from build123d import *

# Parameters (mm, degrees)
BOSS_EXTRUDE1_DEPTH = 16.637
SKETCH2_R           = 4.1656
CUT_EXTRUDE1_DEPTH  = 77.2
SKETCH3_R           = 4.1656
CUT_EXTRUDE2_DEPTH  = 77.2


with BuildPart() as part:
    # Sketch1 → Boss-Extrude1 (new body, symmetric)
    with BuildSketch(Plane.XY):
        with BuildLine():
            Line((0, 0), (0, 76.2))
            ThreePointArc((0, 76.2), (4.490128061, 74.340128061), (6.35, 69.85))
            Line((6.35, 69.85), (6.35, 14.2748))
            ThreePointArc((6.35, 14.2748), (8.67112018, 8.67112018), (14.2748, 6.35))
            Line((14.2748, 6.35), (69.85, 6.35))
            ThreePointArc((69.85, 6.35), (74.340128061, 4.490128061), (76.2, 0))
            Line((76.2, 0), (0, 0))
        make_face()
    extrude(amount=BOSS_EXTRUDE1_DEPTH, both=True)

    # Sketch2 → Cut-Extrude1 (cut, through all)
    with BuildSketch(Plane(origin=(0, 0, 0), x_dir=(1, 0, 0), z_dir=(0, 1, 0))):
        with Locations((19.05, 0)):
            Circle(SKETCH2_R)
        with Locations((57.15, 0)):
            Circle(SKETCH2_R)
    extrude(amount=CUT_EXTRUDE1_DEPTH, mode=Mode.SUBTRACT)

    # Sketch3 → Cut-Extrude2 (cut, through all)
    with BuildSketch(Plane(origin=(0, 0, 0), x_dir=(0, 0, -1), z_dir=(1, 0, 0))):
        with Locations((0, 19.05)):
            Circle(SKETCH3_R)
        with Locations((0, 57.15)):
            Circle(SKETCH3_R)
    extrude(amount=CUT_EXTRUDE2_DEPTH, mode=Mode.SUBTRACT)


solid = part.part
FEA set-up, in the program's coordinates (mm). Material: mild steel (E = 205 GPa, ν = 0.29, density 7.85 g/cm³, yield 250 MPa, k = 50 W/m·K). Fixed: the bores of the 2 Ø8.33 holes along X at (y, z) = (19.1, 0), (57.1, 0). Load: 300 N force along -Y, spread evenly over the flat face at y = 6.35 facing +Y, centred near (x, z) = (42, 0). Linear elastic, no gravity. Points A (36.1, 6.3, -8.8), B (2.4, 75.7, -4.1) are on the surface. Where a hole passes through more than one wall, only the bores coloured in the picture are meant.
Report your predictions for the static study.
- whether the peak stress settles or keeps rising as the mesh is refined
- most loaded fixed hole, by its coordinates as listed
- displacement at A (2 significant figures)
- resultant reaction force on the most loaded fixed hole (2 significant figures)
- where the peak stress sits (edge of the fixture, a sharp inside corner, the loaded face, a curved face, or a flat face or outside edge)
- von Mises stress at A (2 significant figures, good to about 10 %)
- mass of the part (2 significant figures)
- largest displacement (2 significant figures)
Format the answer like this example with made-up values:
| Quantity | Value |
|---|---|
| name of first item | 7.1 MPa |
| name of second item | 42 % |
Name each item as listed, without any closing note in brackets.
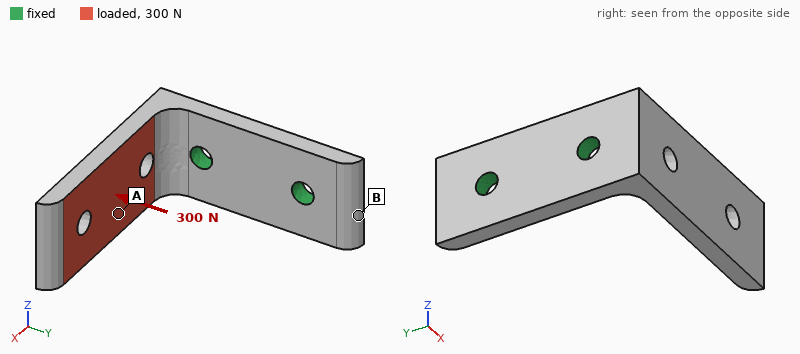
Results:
| Quantity | Value |
|---|---|
| whether the peak stress settles or keeps rising as the mesh is refined | keeps rising |
| most loaded fixed hole, by its coordinates as listed | (19.1, 0) |
| displacement at A | 0.048 mm |
| resultant reaction force on the most loaded fixed hole | 290 N |
| where the peak stress sits | edge of the fixture |
| von Mises stress at A | 14 MPa |
| mass of the part | 230 g |
| largest displacement | 0.14 mm |
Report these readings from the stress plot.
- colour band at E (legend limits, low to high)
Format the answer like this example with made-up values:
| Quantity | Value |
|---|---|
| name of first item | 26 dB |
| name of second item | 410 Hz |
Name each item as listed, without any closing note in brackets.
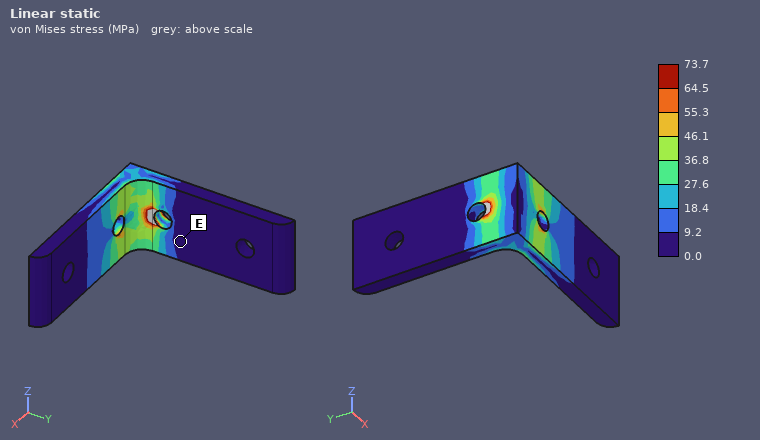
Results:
| Quantity | Value |
|---|---|
| colour band at E | 0.0 to 9.2 MPa |
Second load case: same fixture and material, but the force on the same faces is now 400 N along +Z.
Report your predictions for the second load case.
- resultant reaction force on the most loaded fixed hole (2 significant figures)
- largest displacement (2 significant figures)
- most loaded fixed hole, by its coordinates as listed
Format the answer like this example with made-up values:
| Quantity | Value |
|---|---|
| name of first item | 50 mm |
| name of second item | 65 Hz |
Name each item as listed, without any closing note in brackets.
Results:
| Quantity | Value |
|---|---|
| resultant reaction force on the most loaded fixed hole | 470 N |
| largest displacement | 51 µm |
| most loaded fixed hole, by its coordinates as listed | (19.1, 0) |
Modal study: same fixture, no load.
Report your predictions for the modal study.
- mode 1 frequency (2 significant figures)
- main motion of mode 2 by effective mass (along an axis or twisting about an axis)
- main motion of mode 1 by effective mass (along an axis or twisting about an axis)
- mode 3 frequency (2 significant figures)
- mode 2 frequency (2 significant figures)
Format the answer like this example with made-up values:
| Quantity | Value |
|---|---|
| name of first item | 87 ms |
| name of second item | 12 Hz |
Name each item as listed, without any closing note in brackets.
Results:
| Quantity | Value |
|---|---|
| mode 1 frequency | 890 Hz |
| main motion of mode 2 by effective mass | along Z |
| main motion of mode 1 by effective mass | along Y |
| mode 3 frequency | 4300 Hz |
| mode 2 frequency | 1700 Hz |
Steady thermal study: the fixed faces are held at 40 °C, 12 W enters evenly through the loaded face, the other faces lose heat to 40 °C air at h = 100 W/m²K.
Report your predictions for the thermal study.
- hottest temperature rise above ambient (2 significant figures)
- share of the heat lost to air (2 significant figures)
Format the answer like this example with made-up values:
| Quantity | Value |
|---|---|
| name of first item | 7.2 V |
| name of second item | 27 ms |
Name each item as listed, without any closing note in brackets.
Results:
| Quantity | Value |
|---|---|
| hottest temperature rise above ambient | 22 K |
| share of the heat lost to air | 63 % |
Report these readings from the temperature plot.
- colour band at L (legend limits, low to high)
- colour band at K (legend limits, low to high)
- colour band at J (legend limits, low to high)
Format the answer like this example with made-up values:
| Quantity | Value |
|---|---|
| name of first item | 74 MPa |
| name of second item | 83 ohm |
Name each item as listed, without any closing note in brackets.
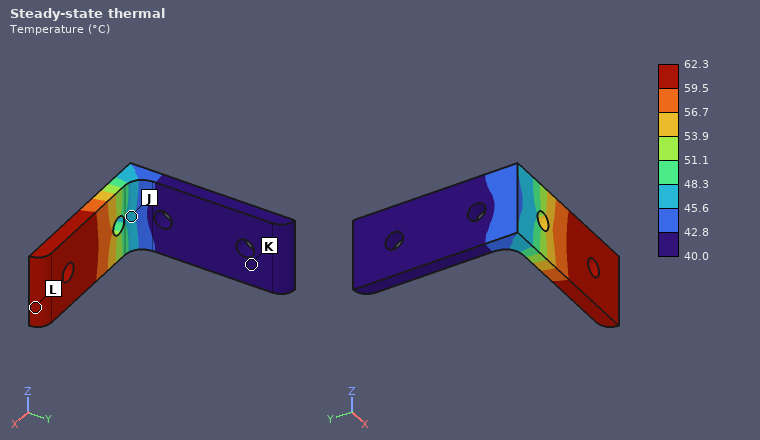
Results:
| Quantity | Value |
|---|---|
| colour band at L | 59.5 to 62.3 °C |
| colour band at K | 40.0 to 42.8 °C |
| colour band at J | 45.6 to 48.3 °C |
